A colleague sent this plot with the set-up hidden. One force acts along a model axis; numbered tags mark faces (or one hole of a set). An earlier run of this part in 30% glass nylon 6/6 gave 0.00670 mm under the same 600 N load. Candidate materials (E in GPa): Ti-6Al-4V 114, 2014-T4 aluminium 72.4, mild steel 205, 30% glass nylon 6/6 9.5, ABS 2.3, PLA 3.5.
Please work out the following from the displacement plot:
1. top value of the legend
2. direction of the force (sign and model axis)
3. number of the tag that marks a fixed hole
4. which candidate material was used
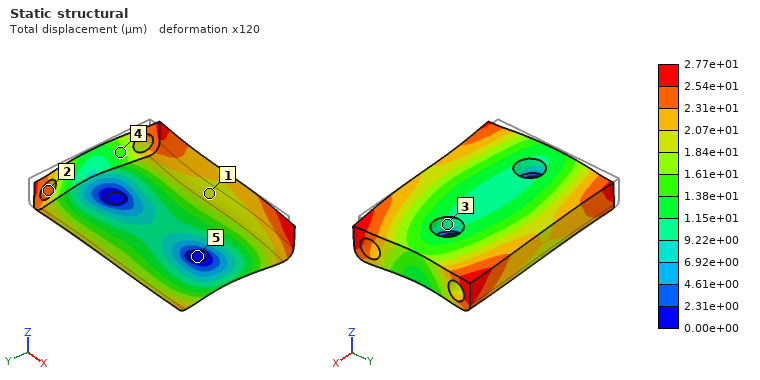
2.77e+01 µm
+X
5
ABS
